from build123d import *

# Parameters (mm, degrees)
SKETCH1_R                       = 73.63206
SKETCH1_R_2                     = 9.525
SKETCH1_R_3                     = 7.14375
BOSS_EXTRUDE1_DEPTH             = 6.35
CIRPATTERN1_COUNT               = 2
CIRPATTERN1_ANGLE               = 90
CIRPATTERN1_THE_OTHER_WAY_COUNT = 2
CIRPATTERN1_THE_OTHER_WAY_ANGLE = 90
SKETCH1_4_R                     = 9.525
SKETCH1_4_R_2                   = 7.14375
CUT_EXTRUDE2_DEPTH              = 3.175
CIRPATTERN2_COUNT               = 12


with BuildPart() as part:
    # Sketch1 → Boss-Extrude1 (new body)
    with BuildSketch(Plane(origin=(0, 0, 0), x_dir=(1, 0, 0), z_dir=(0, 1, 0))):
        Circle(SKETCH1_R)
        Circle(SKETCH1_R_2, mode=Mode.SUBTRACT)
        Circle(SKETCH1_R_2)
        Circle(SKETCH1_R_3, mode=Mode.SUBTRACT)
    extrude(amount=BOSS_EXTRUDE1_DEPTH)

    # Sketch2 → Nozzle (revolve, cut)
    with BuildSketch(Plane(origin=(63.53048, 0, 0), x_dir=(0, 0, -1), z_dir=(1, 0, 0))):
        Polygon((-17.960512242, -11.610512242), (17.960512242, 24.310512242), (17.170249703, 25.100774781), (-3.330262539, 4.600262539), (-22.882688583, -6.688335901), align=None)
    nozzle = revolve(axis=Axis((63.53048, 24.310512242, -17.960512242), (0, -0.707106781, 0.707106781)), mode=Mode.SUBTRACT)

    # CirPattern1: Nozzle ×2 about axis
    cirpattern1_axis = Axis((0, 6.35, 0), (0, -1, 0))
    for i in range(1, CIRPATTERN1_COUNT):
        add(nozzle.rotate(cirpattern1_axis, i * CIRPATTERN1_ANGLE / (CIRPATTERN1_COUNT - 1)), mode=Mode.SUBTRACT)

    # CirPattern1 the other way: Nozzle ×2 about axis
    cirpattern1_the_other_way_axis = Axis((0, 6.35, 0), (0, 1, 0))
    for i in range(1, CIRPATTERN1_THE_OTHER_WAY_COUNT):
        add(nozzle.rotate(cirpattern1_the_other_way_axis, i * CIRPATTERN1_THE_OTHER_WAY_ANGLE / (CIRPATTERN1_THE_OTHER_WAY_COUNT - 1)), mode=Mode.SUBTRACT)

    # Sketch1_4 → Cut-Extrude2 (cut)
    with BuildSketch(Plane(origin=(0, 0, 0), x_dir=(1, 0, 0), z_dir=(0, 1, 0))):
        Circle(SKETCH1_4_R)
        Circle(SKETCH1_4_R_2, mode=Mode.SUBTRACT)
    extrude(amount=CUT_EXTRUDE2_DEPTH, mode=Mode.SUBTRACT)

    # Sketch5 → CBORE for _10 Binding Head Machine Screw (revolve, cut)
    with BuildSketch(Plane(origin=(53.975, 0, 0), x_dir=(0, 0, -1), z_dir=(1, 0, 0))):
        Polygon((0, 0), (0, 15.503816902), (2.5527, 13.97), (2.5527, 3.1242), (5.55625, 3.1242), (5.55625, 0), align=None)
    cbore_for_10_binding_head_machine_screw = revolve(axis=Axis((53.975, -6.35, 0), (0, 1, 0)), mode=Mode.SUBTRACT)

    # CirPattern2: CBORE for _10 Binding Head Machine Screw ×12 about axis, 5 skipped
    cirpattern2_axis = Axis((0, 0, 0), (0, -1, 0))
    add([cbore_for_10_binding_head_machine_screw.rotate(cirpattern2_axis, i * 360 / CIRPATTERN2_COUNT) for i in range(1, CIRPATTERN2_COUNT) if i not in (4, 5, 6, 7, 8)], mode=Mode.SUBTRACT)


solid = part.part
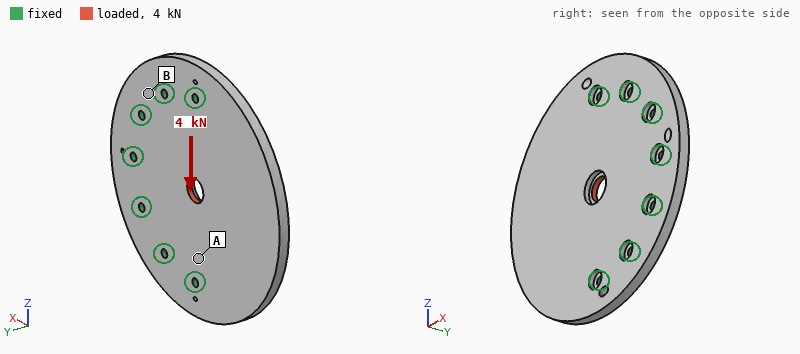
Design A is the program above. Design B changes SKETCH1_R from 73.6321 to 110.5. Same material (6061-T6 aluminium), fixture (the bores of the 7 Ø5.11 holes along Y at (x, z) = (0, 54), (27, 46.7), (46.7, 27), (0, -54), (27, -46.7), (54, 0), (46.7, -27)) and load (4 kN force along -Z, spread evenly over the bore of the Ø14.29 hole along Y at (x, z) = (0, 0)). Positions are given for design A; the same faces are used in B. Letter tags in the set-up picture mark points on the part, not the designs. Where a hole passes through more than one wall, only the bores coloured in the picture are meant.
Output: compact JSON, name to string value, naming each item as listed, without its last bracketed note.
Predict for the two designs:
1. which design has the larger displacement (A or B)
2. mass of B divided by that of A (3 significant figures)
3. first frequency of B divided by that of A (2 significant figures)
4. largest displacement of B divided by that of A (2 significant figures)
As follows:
{"which design has the larger displacement": "B", "mass of B divided by that of A": "2.30", "first frequency of B divided by that of A": "0.52", "largest displacement of B divided by that of A": "1.3"}
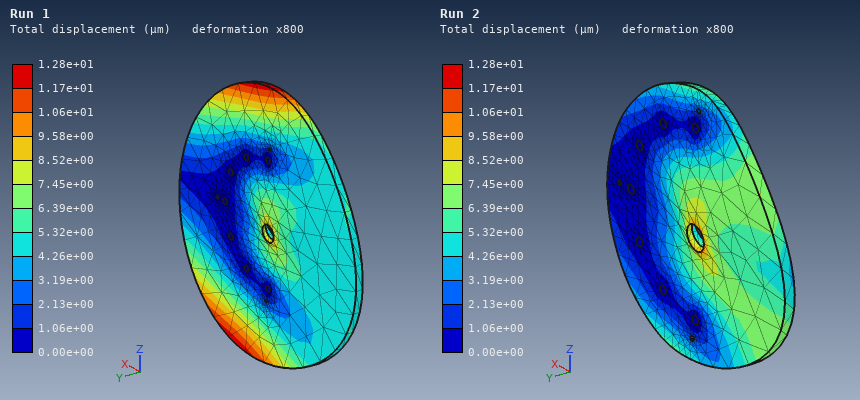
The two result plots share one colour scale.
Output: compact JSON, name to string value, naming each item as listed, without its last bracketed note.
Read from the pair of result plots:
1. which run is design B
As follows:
{"which run is design B": "Run 1"}
